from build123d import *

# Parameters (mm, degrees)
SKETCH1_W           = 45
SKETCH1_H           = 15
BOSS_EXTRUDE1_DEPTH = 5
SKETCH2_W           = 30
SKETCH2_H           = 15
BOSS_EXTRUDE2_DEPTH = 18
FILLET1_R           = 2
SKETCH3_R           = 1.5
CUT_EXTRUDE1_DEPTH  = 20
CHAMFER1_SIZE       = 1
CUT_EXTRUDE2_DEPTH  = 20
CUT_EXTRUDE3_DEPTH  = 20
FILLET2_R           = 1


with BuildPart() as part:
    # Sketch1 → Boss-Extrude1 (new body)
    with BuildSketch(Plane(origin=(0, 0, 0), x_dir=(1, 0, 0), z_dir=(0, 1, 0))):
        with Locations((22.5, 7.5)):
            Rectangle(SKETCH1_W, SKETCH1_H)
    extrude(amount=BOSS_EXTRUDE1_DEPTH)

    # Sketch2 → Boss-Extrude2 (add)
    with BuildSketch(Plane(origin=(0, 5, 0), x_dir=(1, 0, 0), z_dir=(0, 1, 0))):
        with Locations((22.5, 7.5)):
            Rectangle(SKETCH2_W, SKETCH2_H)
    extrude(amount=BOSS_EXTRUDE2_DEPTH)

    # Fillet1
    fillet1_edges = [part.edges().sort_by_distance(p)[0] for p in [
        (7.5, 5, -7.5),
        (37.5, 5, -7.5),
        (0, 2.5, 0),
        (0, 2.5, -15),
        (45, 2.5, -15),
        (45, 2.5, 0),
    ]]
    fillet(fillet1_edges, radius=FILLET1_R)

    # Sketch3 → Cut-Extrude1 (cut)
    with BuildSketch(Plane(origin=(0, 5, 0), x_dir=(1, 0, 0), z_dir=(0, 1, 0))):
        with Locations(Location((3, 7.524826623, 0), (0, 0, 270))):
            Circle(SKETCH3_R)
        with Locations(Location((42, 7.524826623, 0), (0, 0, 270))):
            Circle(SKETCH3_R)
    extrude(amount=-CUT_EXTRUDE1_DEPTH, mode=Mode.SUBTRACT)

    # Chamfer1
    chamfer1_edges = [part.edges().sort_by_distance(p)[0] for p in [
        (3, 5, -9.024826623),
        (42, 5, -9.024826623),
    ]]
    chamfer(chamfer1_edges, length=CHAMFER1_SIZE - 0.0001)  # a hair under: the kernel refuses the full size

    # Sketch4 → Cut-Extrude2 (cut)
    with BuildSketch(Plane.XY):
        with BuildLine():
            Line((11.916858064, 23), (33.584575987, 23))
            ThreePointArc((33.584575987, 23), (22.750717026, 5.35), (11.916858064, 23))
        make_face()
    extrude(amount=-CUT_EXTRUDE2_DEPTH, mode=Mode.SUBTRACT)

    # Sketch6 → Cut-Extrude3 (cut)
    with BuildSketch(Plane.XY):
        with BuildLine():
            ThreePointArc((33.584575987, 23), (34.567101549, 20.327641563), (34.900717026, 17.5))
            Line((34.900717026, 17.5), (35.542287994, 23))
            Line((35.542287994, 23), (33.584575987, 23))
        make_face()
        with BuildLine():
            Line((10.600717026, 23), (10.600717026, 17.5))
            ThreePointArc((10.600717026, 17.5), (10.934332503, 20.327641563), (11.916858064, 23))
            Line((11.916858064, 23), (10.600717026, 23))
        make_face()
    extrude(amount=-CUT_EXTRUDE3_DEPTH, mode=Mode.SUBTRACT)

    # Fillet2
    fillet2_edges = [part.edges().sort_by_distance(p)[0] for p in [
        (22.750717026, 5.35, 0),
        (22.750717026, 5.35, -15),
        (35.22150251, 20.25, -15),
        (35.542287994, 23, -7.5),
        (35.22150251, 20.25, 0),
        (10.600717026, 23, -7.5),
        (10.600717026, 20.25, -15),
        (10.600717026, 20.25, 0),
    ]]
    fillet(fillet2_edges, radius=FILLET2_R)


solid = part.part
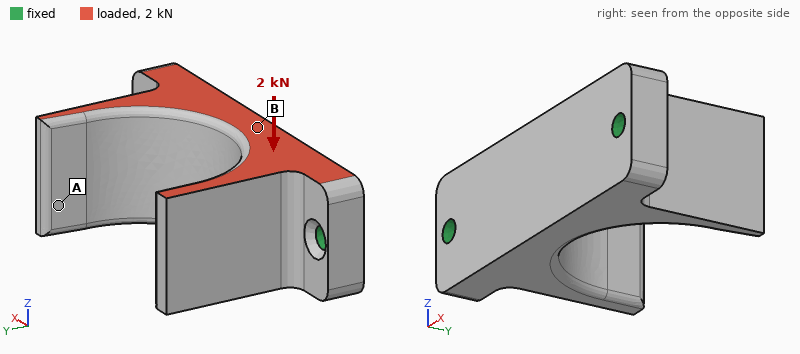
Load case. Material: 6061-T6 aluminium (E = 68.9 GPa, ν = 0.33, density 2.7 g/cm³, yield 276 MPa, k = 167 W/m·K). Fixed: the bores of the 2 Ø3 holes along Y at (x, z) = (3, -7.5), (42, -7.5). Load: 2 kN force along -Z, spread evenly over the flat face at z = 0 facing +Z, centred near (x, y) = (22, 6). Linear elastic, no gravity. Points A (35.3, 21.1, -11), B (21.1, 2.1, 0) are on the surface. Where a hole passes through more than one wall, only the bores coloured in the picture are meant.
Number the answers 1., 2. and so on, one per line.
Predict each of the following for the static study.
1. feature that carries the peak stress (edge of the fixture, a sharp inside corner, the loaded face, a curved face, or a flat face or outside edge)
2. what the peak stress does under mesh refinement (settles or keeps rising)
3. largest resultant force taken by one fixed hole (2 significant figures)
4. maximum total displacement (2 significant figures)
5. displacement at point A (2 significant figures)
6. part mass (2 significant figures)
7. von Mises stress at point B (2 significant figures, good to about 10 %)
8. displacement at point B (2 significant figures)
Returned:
1. edge of the fixture
2. keeps rising
3. 1.0 kN
4. 52 µm
5. 42 µm
6. 16 g
7. 27 MPa
8. 17 µm
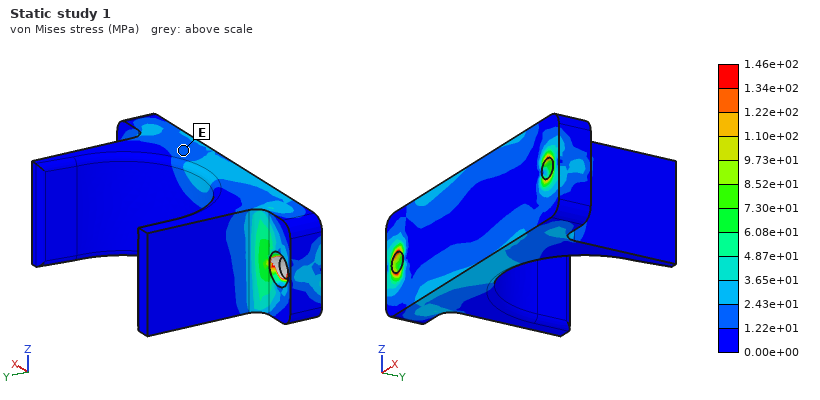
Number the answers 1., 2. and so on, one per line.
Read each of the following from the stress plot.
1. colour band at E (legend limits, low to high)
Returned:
1. 1.22e+01 to 2.43e+01 MPa
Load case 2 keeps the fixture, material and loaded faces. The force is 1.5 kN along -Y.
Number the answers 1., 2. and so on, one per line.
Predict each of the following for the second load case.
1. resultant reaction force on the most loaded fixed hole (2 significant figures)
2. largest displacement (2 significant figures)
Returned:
1. 830 N
2. 75 µm
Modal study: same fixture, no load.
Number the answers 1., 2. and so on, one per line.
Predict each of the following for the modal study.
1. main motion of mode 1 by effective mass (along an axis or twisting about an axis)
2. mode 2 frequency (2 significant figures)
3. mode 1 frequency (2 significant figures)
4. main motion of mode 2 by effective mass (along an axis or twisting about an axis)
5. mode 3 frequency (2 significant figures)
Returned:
1. along Z
2. 9600 Hz
3. 9100 Hz
4. along Y
5. 15 kHz
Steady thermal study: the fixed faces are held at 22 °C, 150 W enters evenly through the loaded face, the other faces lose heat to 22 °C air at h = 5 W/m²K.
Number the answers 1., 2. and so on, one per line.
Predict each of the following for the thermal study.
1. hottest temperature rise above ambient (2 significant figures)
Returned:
1. 71 K
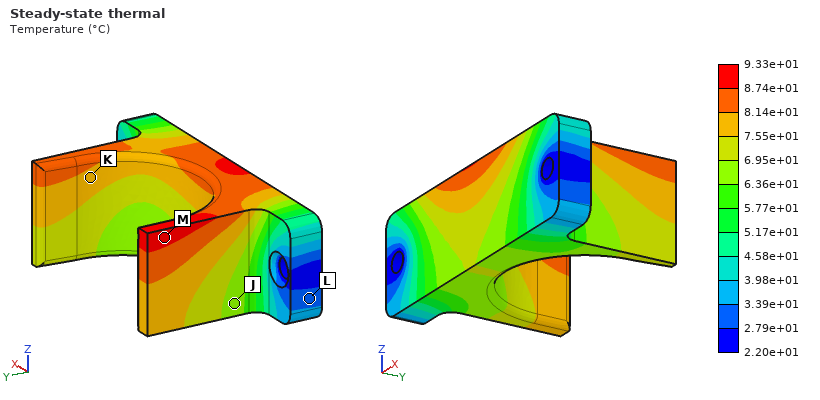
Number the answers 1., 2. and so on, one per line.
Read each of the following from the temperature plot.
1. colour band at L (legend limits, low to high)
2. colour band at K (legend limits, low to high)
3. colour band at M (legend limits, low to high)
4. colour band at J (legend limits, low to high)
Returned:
1. 2.79e+01 to 3.39e+01 °C
2. 7.55e+01 to 8.14e+01 °C
3. 8.74e+01 to 9.33e+01 °C
4. 6.36e+01 to 6.95e+01 °C
